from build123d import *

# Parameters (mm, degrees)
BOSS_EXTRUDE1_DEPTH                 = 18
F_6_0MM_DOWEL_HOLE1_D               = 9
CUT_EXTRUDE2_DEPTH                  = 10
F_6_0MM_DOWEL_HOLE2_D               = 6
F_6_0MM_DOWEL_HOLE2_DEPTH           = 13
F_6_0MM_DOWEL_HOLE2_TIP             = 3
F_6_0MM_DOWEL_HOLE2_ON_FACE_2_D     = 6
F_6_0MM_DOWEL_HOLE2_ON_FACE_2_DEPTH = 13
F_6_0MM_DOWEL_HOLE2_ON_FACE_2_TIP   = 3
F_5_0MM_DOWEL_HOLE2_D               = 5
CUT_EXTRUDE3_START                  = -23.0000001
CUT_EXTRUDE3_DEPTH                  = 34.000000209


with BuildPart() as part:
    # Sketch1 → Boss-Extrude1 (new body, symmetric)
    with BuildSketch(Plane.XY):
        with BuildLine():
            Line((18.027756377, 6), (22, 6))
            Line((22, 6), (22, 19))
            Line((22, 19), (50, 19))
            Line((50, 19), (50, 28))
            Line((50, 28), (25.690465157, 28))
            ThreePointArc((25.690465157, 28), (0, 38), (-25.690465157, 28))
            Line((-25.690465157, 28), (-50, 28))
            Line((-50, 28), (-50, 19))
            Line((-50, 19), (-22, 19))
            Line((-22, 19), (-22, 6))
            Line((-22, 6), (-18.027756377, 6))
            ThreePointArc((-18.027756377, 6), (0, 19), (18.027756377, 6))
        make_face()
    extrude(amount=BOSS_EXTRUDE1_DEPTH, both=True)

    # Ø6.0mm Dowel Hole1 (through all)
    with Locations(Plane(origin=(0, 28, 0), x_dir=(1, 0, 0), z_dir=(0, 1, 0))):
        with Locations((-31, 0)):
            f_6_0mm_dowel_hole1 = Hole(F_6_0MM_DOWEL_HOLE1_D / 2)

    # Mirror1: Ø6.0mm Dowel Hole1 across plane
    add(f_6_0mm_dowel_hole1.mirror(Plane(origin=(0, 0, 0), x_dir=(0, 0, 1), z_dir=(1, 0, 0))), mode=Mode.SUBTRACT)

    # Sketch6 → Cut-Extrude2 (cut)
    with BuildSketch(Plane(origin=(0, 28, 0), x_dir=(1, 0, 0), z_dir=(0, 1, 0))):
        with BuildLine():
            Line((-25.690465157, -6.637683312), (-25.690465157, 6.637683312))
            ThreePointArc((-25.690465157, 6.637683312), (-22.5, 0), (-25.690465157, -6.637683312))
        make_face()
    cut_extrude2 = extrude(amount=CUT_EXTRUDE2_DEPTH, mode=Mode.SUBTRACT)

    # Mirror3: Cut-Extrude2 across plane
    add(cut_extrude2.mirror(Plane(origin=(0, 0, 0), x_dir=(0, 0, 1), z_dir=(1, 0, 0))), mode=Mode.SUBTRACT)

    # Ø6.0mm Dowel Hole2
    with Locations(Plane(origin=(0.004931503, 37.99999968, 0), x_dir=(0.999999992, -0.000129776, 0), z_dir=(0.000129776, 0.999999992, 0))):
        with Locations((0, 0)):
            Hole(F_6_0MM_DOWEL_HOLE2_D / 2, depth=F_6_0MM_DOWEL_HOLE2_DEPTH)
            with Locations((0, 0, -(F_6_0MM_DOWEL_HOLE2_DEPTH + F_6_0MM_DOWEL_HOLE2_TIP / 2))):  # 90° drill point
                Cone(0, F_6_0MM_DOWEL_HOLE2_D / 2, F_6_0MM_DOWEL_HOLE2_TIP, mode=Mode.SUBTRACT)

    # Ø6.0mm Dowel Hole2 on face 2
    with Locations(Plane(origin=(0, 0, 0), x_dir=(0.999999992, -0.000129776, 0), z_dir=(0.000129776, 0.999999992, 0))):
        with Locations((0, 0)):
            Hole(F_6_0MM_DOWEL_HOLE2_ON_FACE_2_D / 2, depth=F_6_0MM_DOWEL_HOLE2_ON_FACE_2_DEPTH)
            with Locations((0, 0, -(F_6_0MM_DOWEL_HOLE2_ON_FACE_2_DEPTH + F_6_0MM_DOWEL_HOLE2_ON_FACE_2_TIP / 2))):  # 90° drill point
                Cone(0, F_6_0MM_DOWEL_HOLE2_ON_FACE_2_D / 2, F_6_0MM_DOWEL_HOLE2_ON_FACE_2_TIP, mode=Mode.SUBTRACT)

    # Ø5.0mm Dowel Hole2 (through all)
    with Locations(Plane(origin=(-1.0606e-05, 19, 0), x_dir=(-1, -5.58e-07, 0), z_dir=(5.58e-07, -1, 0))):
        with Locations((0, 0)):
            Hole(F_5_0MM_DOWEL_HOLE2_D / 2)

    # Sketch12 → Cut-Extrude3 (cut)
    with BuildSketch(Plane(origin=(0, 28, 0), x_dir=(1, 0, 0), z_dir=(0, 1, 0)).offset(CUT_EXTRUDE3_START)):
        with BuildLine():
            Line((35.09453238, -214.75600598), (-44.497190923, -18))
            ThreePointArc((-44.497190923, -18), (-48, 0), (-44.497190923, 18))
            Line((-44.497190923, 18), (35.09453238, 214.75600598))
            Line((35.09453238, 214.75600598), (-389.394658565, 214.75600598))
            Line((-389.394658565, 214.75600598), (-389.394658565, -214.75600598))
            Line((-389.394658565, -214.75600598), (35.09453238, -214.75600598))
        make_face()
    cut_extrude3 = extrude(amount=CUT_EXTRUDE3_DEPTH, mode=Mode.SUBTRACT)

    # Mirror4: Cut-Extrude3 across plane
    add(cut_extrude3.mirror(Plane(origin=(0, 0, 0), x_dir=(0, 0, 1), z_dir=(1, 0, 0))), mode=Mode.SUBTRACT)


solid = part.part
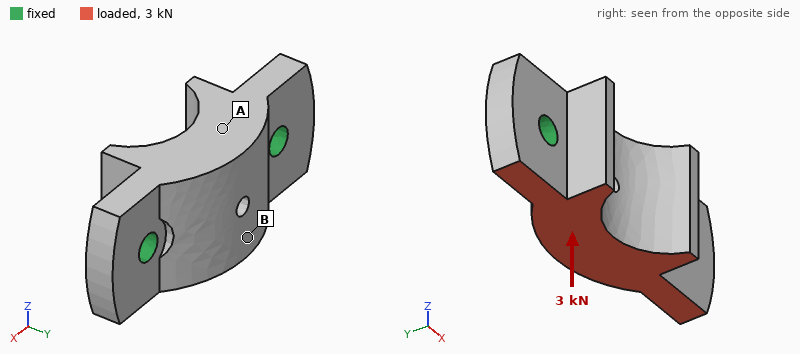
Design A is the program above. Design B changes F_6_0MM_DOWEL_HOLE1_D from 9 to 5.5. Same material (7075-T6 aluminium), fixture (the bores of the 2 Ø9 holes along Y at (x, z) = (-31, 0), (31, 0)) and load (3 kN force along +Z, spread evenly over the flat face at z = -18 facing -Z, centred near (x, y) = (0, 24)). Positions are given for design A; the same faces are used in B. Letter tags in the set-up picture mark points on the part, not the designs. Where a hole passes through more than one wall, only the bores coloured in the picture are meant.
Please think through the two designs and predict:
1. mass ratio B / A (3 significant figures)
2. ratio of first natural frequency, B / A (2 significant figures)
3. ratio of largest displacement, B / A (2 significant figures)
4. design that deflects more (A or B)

1.01
0.79
1.3
B
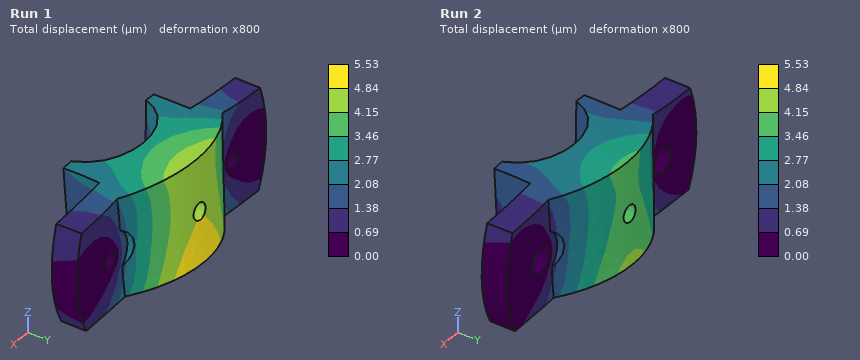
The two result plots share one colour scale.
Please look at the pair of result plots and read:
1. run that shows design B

Run 1
